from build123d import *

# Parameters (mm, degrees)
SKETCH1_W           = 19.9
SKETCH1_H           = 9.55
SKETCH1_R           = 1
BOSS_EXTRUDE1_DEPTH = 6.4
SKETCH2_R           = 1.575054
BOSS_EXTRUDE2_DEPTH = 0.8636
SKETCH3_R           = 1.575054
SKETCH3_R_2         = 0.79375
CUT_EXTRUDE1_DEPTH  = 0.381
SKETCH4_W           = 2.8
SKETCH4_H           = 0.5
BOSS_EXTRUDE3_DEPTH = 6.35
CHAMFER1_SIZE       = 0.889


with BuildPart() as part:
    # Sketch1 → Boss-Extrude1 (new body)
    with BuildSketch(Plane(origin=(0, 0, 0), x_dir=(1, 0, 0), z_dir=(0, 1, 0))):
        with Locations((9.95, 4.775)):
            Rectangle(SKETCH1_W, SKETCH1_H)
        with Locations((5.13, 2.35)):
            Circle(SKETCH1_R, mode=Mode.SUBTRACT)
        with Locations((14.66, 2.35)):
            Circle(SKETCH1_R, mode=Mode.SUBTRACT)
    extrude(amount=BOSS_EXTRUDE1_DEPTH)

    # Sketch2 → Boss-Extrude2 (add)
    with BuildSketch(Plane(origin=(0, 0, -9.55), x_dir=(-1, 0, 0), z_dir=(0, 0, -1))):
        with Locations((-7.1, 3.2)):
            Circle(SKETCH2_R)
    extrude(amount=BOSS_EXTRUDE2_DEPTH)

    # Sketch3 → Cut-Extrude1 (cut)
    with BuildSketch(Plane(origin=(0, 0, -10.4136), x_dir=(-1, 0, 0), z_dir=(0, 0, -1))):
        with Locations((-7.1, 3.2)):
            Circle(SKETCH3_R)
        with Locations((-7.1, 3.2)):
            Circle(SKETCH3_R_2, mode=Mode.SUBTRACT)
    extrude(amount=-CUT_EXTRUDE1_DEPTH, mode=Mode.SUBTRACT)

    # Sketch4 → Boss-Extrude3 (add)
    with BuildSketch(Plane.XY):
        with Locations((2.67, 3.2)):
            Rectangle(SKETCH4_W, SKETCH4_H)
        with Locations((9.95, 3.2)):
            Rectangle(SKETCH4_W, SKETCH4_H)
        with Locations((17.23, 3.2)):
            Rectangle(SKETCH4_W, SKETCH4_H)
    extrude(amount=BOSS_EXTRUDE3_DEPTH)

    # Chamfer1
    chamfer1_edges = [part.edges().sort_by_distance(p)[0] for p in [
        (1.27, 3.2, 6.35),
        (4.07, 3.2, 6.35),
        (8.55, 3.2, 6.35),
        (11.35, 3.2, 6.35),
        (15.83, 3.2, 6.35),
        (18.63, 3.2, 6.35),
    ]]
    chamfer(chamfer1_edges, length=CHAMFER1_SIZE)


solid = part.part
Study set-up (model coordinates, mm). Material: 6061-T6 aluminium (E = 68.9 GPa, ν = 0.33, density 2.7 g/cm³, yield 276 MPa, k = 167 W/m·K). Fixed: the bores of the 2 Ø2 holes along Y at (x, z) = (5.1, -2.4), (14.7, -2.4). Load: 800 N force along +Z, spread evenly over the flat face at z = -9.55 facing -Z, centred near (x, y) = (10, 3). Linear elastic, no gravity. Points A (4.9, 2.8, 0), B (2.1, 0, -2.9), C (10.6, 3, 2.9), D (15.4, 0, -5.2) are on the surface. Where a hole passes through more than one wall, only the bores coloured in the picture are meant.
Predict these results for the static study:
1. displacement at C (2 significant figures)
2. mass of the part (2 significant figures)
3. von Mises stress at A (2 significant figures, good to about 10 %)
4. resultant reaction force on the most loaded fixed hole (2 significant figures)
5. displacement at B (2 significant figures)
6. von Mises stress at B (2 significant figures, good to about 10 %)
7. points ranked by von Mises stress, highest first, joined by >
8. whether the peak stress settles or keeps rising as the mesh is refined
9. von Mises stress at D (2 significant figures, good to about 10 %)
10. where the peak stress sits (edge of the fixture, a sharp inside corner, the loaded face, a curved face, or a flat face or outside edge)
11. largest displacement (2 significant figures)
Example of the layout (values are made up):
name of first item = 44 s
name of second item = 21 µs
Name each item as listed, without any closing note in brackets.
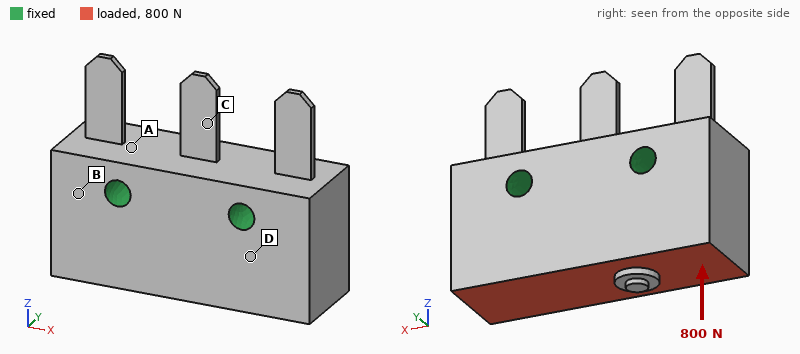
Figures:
displacement at C = 0.29 µm
mass of the part = 3.3 g
von Mises stress at A = 8.5 MPa
resultant reaction force on the most loaded fixed hole = 420 N
displacement at B = 0.57 µm
von Mises stress at B = 4.1 MPa
points ranked by von Mises stress, highest first, joined by > = D > A > B > C
whether the peak stress settles or keeps rising as the mesh is refined = keeps rising
von Mises stress at D = 11 MPa
where the peak stress sits = edge of the fixture
largest displacement = 1.7 µm
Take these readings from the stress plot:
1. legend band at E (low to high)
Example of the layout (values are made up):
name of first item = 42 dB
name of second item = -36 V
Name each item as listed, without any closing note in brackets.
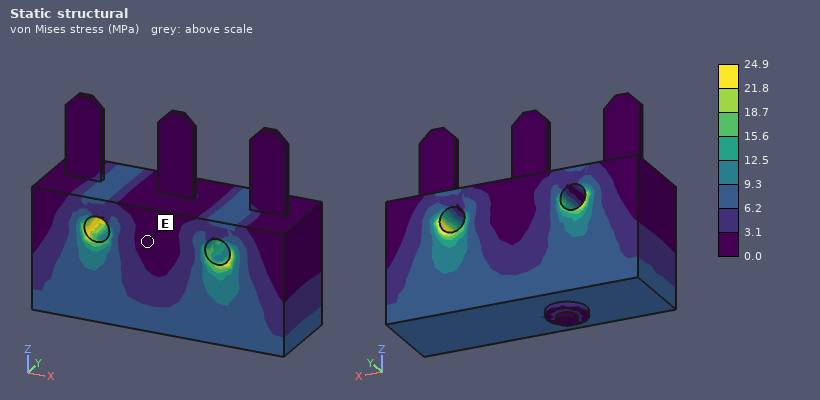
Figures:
legend band at E = 0.0 to 3.1 MPa
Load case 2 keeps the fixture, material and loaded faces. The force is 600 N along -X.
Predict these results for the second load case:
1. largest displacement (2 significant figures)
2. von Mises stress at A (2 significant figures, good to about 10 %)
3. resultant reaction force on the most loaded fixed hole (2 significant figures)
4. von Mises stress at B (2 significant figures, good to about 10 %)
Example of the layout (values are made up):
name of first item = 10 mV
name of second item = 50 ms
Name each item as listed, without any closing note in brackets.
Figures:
largest displacement = 4.2 µm
von Mises stress at A = 13 MPa
resultant reaction force on the most loaded fixed hole = 470 N
von Mises stress at B = 6.1 MPa
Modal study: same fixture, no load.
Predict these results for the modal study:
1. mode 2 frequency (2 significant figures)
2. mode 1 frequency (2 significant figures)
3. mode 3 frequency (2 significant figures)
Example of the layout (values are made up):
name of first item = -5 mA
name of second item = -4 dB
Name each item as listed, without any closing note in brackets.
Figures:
mode 2 frequency = 11 kHz
mode 1 frequency = 11 kHz
mode 3 frequency = 11 kHz
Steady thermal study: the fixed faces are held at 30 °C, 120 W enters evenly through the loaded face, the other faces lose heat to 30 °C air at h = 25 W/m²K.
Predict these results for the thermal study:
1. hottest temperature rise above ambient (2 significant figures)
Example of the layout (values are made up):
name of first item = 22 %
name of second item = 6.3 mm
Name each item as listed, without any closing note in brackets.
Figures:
hottest temperature rise above ambient = 47 K
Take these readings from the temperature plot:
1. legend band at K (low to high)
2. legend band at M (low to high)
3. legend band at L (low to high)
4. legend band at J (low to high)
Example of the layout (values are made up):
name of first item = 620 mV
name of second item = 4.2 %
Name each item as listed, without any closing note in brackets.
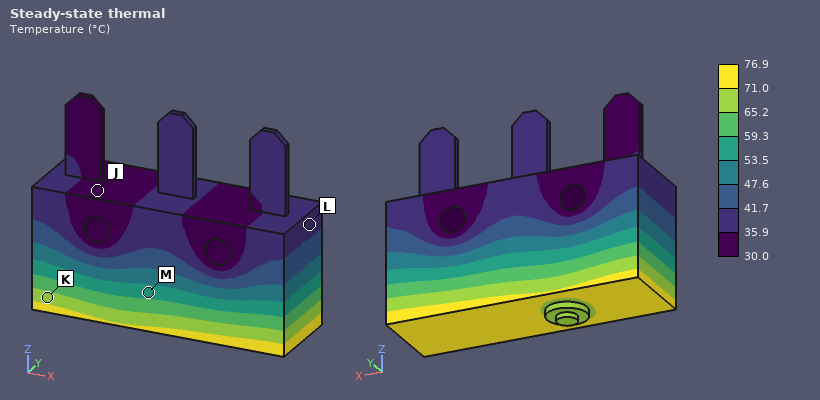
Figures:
legend band at K = 65.2 to 71.0 °C
legend band at M = 53.5 to 59.3 °C
legend band at L = 35.9 to 41.7 °C
legend band at J = 30.0 to 35.9 °C
